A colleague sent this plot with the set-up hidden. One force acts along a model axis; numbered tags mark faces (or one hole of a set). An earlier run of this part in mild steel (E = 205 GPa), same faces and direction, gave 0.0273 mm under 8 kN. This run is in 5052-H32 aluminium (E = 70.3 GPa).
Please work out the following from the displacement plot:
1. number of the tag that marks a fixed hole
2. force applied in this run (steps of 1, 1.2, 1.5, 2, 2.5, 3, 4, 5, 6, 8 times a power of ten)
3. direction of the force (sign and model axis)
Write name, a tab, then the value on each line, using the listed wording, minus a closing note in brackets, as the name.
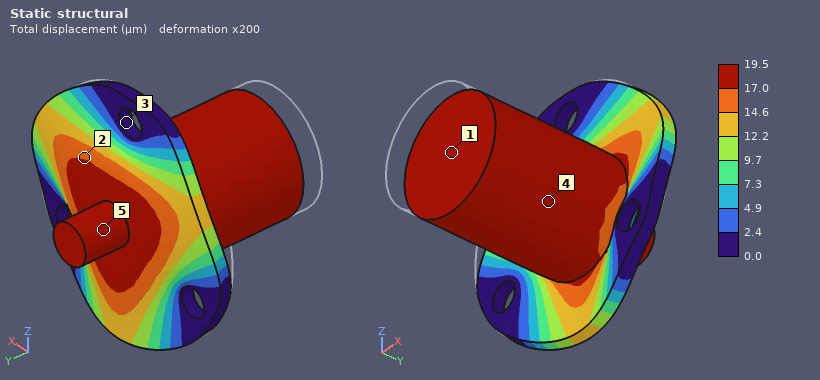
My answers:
number of the tag that marks a fixed hole	3
force applied in this run	2 kN
direction of the force	+Y
